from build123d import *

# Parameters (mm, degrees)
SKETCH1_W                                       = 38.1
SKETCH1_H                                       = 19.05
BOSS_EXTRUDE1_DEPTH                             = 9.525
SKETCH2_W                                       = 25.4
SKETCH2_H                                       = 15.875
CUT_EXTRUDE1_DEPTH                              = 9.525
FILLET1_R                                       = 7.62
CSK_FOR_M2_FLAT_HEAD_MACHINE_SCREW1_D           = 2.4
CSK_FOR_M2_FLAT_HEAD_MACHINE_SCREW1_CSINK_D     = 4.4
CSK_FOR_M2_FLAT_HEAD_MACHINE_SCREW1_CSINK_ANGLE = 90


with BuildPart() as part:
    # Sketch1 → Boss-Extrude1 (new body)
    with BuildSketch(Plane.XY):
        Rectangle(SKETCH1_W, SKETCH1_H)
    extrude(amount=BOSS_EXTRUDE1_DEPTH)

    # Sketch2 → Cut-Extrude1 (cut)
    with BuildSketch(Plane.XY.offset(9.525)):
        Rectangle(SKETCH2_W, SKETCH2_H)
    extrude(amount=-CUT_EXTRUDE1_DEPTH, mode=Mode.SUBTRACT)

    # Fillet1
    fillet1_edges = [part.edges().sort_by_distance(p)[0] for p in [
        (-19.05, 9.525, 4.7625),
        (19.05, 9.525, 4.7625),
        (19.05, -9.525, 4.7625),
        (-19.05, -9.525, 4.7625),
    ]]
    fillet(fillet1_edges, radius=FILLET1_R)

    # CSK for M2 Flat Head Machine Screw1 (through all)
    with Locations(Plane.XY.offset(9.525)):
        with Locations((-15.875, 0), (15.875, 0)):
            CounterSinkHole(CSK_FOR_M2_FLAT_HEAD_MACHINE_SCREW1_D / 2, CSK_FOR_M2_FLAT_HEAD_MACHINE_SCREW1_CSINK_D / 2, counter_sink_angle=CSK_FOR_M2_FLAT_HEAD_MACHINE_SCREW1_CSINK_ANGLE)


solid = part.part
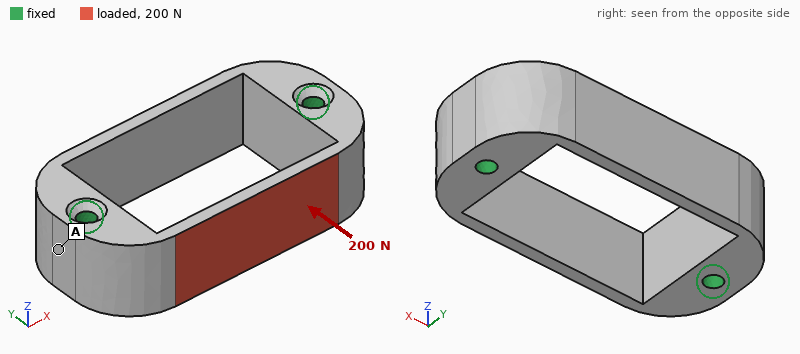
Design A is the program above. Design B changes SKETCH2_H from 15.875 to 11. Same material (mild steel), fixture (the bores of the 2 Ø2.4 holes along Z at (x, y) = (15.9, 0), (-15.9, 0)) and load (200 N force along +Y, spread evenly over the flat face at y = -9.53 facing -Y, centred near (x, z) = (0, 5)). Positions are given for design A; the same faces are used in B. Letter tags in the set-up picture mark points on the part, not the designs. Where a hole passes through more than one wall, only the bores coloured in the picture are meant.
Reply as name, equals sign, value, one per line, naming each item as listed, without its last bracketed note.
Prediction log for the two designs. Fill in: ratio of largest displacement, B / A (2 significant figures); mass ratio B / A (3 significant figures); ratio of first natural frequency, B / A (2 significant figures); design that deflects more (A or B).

ratio of largest displacement, B / A = 0.11
mass ratio B / A = 1.47
ratio of first natural frequency, B / A = 1.8
design that deflects more = A
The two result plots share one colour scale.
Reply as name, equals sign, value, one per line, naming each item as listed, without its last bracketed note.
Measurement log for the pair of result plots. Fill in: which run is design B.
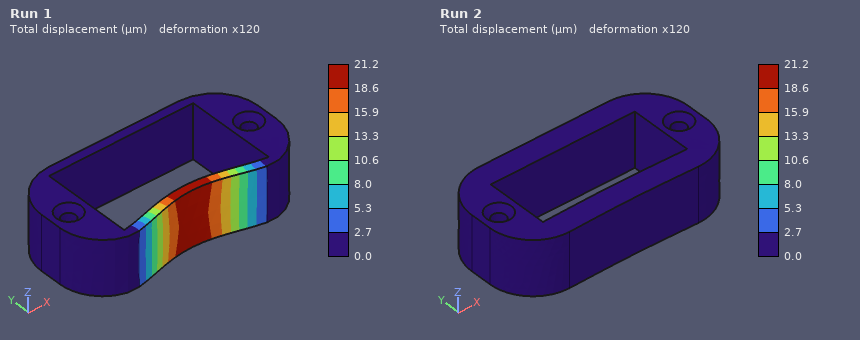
which run is design B = Run 2
